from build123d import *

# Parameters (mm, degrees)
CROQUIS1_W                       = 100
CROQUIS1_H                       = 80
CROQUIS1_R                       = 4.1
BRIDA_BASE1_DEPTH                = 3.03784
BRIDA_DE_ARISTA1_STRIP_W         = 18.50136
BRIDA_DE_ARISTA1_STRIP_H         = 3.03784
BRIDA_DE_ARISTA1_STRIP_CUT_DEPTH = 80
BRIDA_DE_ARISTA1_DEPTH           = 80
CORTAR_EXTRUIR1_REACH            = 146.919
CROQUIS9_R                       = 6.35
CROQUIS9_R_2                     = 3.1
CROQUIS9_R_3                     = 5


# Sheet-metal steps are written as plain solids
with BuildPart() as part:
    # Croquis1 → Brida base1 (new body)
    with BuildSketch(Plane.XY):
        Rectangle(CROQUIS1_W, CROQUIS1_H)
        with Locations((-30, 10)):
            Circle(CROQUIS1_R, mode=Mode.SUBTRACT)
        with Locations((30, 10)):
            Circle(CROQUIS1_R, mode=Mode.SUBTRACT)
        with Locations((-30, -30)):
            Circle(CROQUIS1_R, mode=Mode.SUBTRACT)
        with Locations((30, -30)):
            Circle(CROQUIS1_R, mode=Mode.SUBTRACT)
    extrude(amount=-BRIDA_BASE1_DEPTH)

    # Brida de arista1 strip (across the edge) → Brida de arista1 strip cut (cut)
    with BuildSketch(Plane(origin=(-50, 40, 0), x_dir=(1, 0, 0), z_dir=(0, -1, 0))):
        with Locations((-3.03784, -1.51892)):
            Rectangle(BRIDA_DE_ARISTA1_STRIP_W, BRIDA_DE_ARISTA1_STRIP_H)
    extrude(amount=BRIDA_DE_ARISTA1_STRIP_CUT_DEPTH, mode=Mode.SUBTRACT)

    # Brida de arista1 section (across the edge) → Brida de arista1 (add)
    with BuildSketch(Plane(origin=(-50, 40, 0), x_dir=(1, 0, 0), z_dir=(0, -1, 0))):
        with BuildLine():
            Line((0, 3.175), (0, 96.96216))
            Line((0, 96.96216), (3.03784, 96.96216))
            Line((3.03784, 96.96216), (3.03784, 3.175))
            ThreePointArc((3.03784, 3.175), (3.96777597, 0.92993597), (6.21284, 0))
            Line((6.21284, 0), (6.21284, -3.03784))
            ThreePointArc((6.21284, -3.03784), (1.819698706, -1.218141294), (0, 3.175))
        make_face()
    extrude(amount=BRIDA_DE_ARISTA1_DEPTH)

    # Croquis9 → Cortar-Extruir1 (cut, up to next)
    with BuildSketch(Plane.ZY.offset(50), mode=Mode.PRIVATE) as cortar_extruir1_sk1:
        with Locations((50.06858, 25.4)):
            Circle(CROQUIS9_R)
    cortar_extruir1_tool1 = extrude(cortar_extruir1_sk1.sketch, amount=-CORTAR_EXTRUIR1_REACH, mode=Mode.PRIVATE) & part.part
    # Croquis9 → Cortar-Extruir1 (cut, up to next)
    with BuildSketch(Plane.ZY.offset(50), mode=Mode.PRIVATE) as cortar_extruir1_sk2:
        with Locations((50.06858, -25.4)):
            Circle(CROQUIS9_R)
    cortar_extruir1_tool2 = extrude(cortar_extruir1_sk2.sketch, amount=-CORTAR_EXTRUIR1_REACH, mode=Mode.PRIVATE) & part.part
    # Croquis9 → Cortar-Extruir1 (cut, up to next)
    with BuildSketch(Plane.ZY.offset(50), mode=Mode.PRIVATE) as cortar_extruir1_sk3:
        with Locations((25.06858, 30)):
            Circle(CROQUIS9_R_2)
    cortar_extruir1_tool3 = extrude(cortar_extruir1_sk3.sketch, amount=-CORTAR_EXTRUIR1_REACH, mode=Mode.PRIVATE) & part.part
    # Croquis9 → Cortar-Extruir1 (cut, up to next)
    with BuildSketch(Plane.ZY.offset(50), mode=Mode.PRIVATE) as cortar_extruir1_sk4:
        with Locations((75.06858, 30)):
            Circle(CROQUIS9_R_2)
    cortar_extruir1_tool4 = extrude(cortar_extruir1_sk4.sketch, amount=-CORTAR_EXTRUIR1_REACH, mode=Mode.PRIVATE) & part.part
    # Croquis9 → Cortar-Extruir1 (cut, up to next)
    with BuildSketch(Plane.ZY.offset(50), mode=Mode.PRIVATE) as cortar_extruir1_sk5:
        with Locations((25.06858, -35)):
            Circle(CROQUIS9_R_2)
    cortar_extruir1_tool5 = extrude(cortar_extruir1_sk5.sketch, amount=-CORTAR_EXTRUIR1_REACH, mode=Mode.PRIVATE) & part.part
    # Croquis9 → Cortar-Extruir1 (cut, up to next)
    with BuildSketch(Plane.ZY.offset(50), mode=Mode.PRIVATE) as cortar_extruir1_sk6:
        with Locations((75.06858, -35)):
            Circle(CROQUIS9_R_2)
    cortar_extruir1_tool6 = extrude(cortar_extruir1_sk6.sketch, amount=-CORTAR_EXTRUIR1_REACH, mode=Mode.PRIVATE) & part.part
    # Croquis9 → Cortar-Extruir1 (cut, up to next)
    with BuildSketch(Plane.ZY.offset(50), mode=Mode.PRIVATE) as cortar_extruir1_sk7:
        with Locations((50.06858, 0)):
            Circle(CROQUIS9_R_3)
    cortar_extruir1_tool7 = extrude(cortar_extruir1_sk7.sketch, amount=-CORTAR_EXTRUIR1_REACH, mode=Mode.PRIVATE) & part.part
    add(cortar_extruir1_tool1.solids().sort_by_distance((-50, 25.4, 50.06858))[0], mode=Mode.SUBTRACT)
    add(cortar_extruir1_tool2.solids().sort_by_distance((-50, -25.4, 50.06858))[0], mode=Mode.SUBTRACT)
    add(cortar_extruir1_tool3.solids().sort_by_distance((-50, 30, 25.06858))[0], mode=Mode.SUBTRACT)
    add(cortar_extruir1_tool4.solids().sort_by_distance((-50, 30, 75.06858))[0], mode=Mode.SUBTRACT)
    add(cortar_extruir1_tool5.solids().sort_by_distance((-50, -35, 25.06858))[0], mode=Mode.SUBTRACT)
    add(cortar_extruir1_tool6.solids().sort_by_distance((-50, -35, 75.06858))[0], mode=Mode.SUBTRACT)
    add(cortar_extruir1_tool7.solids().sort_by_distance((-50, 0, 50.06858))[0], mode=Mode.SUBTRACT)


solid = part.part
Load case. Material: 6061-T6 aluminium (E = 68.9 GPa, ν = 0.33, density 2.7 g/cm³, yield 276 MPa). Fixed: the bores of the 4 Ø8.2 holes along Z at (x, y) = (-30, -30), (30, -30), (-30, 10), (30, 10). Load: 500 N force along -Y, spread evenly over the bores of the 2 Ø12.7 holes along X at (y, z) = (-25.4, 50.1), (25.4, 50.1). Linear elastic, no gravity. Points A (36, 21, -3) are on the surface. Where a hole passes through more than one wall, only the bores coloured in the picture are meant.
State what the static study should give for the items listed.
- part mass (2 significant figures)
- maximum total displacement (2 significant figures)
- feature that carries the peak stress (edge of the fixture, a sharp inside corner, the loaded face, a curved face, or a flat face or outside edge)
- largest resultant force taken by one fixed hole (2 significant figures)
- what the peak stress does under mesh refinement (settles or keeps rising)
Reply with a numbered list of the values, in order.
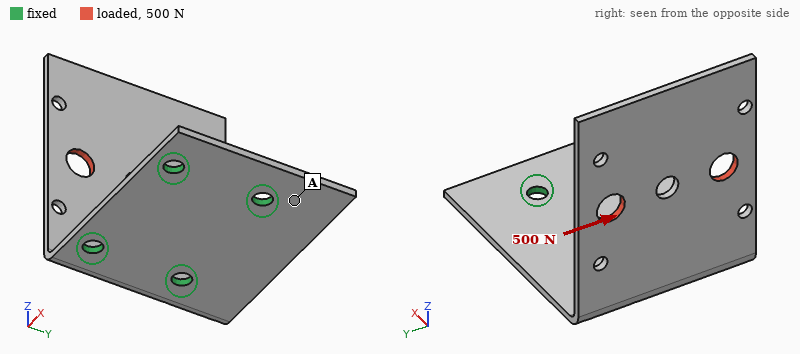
1. 120 g
2. 0.62 mm
3. edge of the fixture
4. 650 N
5. keeps rising
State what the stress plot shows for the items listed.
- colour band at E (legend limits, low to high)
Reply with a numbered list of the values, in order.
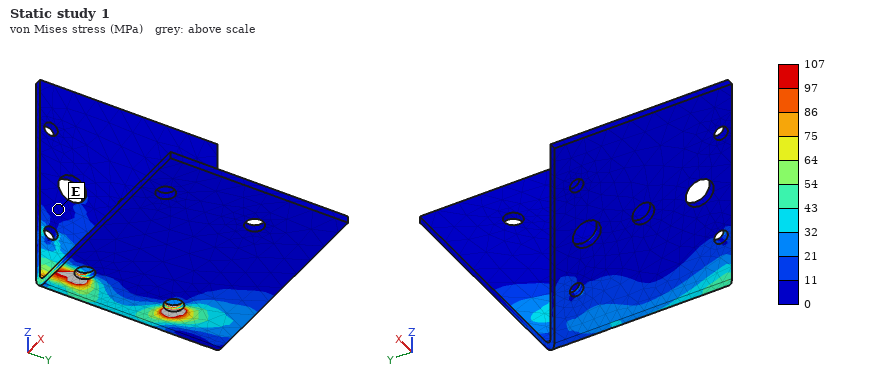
1. 0 to 11 MPa
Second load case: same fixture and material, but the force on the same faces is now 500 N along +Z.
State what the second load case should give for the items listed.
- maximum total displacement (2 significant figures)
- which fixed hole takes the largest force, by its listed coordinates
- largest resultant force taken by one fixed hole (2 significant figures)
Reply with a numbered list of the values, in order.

1. 0.60 mm
2. (-30, 10)
3. 370 N
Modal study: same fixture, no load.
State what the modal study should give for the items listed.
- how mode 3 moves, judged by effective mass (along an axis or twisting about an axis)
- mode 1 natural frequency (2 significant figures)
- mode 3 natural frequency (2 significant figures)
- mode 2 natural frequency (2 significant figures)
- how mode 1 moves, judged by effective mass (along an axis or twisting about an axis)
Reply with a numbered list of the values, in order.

1. along Y
2. 210 Hz
3. 870 Hz
4. 620 Hz
5. along X
